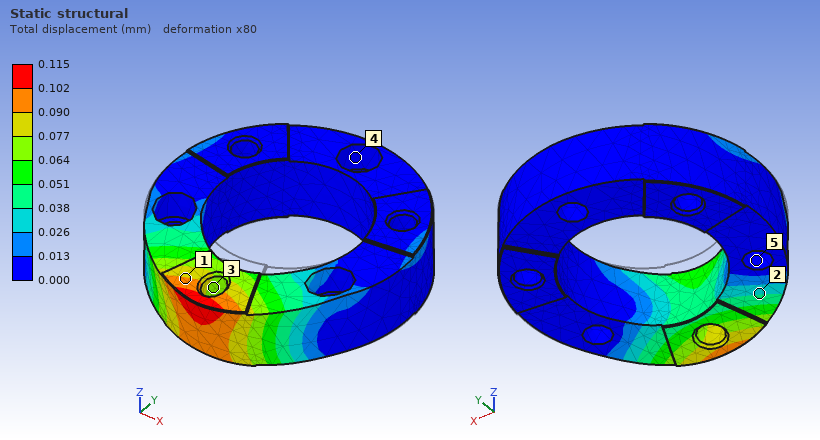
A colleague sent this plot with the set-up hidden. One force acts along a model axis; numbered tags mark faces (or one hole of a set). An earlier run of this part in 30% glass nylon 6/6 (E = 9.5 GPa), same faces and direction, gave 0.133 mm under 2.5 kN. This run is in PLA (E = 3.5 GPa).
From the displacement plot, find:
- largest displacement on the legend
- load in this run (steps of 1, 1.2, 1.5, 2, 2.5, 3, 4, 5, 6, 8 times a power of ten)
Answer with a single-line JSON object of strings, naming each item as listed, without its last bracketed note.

{"largest displacement on the legend": "0.115 mm", "load in this run": "800 N"}
